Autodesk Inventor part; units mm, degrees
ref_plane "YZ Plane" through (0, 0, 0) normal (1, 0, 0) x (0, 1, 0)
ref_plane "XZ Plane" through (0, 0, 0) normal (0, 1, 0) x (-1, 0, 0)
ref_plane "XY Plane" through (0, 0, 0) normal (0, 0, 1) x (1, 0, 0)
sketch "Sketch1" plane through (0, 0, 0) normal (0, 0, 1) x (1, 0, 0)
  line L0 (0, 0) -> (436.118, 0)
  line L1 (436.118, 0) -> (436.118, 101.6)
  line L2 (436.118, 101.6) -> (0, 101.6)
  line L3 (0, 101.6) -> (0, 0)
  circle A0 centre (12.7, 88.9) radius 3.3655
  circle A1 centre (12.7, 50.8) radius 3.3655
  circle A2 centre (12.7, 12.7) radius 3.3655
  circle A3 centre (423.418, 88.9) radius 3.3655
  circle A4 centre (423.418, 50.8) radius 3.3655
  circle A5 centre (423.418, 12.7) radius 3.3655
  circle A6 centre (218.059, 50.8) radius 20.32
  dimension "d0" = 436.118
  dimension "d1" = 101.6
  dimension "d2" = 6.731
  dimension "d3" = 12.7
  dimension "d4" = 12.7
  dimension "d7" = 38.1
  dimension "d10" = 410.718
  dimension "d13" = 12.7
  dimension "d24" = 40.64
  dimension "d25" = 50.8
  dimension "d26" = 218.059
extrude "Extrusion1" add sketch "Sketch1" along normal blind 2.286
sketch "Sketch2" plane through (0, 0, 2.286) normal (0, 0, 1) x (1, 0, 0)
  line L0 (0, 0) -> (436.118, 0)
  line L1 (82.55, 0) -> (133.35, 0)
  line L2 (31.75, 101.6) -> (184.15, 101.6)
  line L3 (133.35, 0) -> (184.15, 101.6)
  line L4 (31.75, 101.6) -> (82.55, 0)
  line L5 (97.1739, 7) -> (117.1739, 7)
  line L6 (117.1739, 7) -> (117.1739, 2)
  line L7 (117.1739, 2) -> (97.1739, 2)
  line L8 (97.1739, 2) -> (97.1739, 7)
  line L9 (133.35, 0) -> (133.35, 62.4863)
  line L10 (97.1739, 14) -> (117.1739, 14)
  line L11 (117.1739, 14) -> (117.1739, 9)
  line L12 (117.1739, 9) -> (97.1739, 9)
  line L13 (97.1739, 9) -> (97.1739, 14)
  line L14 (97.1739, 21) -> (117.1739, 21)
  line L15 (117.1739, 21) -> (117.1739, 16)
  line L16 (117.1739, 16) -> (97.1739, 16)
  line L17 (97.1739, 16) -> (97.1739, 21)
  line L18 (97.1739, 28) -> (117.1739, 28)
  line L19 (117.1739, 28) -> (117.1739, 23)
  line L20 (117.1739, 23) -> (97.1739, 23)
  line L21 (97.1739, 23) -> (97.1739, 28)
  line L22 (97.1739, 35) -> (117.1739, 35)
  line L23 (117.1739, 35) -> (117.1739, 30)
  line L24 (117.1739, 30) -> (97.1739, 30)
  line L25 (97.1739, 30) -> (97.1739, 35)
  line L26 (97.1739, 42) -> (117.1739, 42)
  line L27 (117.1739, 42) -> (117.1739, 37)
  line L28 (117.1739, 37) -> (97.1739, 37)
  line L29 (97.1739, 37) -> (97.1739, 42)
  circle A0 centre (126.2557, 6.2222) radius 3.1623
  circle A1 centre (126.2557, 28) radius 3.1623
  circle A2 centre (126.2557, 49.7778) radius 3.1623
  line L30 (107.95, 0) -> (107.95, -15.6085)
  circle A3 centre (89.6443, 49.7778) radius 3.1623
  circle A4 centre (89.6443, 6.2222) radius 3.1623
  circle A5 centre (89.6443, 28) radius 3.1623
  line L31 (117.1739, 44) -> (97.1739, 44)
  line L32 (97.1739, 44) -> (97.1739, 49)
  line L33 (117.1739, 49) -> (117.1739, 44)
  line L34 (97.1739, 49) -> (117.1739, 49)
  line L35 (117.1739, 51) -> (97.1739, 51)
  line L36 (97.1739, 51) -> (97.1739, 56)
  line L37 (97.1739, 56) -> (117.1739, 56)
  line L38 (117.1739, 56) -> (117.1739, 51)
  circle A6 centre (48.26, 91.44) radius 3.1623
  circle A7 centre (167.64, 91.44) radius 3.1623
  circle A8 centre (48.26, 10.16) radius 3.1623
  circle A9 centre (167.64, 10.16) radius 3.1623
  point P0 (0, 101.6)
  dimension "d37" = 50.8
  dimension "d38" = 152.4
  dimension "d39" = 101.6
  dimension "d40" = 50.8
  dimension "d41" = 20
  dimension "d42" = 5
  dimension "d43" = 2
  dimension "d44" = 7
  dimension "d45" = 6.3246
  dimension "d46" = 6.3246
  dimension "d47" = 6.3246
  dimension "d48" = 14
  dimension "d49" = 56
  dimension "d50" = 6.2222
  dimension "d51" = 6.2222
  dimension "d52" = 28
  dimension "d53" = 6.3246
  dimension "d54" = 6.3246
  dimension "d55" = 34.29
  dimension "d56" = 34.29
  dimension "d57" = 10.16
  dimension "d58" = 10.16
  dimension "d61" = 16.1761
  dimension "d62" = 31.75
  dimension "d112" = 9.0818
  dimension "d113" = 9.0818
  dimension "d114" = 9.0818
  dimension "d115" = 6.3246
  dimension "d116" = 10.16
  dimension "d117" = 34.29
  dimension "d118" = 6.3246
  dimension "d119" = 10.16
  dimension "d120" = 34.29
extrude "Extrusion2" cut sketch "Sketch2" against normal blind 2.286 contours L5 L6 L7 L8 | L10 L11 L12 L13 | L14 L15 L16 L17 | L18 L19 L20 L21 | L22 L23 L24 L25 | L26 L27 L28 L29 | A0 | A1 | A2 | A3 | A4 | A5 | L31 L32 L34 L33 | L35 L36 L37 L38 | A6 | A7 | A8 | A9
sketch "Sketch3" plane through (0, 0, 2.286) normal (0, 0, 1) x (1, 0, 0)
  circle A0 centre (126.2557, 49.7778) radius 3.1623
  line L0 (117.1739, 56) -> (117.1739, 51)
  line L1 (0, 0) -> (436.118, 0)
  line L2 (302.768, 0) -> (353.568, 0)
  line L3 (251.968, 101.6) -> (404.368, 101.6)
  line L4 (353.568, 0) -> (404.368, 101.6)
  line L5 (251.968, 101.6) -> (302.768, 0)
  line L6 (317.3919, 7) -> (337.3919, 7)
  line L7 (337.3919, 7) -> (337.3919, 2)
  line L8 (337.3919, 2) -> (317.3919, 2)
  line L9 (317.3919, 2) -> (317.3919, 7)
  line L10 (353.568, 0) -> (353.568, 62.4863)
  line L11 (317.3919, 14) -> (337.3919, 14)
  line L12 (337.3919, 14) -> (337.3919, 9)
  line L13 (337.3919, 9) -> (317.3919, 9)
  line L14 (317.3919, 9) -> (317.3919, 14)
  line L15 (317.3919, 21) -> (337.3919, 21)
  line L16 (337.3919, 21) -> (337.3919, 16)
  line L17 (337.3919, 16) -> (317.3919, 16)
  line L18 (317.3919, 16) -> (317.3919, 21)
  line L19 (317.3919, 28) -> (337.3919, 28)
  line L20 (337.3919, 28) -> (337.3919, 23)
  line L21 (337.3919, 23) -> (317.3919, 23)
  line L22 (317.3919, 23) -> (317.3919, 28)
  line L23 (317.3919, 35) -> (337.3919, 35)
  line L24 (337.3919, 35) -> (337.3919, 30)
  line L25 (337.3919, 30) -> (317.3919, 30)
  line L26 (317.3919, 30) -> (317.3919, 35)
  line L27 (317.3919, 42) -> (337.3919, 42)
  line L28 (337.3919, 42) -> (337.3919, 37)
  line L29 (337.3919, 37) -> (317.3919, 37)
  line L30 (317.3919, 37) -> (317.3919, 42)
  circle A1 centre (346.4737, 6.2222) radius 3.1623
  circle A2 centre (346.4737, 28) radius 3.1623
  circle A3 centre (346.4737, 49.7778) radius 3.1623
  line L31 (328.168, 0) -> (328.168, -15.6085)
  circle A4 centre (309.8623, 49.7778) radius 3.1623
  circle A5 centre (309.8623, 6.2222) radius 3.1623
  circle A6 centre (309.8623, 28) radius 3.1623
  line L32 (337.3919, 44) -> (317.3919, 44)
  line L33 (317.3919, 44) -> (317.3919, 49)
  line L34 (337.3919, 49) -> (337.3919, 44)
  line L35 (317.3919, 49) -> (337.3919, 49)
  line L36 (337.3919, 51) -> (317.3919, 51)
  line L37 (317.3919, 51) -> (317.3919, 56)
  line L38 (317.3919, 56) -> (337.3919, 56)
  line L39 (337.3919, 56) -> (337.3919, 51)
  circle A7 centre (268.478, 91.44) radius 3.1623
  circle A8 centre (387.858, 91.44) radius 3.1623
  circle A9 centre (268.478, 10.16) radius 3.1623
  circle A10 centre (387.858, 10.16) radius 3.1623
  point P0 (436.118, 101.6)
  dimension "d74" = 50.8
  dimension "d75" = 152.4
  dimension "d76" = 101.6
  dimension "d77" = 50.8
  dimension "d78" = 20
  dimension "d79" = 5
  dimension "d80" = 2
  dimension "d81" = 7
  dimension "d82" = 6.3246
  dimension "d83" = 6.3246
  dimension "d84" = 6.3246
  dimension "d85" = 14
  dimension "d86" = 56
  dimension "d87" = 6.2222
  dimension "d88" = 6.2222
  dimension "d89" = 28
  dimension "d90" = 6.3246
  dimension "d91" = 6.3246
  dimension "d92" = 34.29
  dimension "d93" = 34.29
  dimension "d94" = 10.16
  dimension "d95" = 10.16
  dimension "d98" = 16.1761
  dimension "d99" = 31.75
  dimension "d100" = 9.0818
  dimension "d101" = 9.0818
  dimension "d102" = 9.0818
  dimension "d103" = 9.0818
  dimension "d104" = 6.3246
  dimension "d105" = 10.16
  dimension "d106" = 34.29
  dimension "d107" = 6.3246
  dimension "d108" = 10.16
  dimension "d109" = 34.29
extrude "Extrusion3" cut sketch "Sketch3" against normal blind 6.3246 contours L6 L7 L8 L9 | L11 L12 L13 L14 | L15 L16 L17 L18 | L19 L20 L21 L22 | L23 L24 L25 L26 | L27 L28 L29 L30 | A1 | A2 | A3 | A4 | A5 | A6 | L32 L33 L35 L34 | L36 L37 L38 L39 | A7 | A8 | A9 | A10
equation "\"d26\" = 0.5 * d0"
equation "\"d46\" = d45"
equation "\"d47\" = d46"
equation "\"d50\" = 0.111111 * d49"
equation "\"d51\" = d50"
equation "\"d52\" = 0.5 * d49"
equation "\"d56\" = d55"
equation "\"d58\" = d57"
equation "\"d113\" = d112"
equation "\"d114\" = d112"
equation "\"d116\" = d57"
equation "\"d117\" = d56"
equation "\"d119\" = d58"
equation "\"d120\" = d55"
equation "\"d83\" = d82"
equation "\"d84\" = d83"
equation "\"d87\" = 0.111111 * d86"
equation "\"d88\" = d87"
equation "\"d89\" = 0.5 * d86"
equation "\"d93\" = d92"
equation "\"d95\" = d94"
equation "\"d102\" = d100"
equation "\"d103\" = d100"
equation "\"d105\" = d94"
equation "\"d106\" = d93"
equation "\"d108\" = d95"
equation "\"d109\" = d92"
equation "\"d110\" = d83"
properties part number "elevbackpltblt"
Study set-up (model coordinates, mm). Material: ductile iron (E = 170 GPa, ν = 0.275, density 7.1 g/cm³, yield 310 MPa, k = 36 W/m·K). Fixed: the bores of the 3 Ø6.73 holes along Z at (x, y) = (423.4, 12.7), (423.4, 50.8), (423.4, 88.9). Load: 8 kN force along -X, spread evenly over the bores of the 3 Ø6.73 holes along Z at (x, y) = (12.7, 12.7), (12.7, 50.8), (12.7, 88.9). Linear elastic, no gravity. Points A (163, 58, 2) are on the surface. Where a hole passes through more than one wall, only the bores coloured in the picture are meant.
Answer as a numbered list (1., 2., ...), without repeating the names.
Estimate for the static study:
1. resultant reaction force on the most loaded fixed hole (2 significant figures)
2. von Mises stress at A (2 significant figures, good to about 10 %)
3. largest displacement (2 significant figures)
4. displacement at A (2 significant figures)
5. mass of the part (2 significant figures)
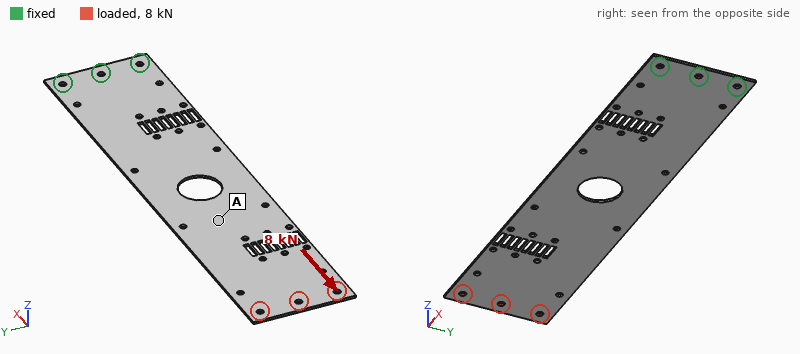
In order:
1. 2.8 kN
2. 25 MPa
3. 0.15 mm
4. 0.078 mm
5. 660 g
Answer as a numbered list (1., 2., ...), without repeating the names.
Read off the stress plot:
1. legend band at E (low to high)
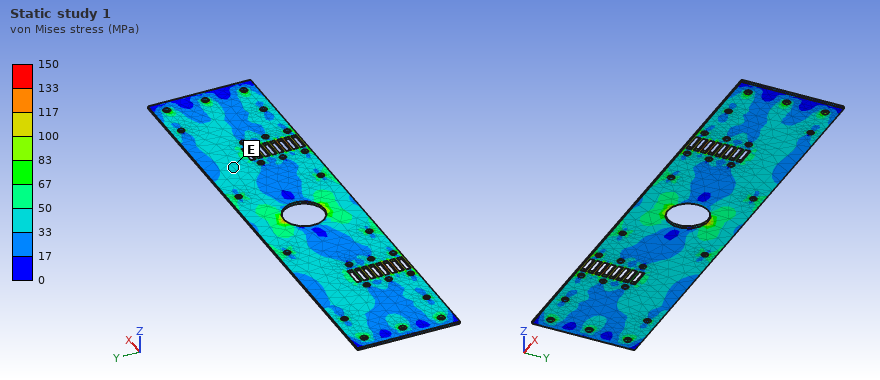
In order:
1. 33 to 50 MPa
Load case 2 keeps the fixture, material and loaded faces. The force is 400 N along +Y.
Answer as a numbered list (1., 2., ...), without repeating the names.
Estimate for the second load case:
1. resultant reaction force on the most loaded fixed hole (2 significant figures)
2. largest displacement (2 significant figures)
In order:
1. 2.1 kN
2. 0.38 mm
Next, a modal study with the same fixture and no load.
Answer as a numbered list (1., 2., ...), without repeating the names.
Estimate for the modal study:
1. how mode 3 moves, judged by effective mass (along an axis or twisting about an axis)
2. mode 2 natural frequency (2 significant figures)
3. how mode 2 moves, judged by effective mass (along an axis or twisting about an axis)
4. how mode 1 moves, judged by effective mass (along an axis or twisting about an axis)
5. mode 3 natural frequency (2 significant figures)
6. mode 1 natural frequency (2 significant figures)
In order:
1. twisting about X
2. 62 Hz
3. along Z
4. along Z
5. 82 Hz
6. 9.8 Hz
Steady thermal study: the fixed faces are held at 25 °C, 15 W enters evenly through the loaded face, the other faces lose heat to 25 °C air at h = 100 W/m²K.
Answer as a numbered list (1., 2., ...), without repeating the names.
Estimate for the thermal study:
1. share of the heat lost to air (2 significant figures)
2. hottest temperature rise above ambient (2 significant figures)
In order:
1. 100 %
2. 31 K
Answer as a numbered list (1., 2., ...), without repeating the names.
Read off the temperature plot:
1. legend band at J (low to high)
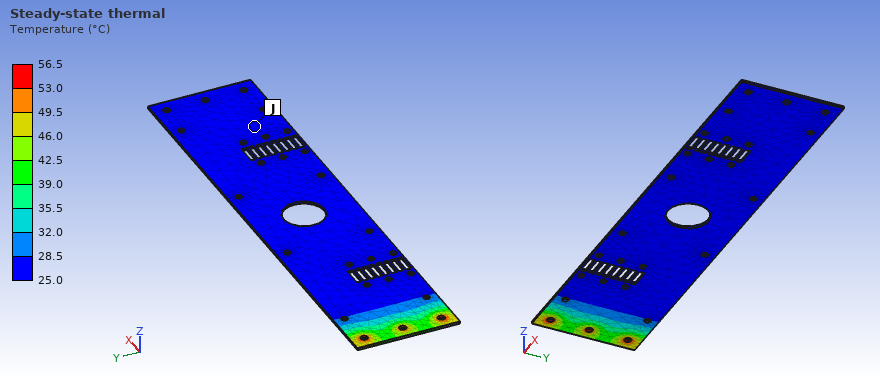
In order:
1. 25.0 to 28.5 °C
